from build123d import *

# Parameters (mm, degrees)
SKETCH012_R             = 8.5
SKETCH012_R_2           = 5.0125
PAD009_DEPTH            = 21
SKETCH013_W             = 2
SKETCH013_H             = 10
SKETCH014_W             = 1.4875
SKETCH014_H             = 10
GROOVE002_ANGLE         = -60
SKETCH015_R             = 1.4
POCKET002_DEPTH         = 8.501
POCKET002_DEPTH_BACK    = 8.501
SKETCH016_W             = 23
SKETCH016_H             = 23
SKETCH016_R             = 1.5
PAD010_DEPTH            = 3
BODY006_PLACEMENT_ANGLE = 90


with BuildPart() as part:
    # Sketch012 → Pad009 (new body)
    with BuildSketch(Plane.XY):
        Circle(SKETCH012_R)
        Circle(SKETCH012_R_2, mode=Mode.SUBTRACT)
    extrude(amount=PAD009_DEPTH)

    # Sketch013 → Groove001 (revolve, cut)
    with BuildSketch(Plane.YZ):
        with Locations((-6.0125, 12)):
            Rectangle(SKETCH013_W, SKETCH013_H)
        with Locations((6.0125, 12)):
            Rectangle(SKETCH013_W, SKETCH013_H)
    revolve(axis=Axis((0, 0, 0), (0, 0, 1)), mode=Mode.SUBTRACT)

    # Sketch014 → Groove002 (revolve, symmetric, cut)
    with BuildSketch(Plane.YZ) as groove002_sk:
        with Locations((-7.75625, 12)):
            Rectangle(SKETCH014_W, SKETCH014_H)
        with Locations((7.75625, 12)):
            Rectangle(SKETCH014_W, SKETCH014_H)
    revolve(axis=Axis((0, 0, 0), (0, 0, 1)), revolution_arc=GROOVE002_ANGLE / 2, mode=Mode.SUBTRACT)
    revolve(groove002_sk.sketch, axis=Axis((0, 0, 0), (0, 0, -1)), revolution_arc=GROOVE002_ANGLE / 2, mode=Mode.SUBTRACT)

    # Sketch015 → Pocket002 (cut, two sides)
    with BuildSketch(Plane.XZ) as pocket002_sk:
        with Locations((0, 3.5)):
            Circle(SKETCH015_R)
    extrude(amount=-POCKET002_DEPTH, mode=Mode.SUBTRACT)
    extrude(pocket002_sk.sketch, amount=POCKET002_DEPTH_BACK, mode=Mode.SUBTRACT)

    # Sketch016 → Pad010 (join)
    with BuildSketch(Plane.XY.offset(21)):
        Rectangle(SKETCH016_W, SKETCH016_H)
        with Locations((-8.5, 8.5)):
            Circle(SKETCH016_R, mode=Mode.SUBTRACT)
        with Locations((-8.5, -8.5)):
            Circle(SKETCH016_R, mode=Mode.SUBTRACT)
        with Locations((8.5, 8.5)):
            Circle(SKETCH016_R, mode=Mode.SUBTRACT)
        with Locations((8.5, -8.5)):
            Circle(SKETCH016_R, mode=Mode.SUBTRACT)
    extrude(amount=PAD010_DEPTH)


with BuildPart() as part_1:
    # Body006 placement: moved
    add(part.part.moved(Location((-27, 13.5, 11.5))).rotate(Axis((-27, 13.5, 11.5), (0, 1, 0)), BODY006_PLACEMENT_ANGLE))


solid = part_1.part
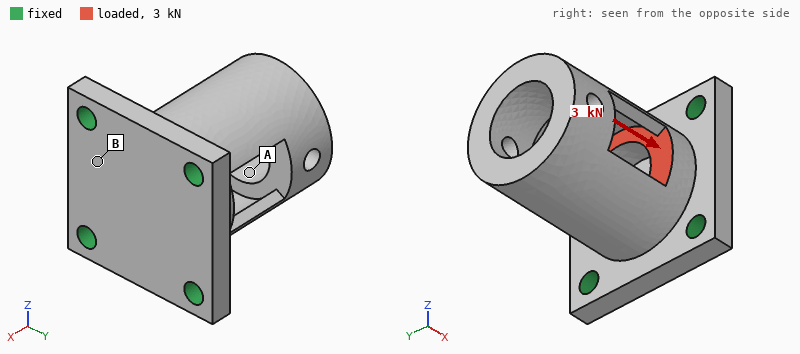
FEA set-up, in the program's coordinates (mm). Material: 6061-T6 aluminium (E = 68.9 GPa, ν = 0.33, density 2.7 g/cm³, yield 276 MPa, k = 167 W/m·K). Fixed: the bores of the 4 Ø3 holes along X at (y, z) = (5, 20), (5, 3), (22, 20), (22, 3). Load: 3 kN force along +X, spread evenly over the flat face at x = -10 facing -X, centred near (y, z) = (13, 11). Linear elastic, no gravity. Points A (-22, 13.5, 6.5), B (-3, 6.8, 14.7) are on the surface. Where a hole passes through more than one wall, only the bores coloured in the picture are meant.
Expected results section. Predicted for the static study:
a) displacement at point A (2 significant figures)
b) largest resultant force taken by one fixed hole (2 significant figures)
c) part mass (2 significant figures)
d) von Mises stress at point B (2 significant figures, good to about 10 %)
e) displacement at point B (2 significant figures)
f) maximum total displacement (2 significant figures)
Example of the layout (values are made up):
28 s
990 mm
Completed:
9.2 µm
790 N
9.6 g
37 MPa
9.7 µm
13 µm
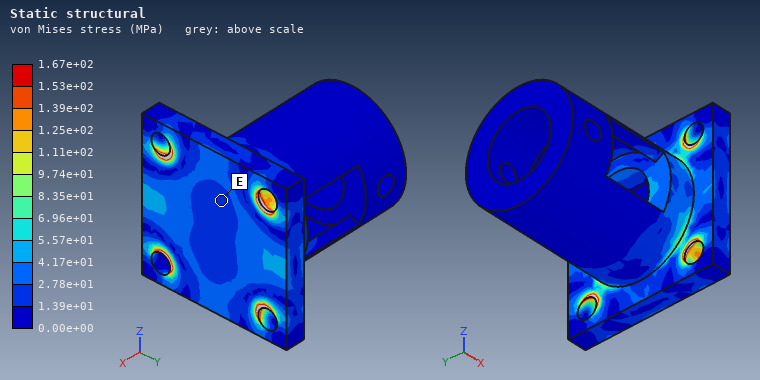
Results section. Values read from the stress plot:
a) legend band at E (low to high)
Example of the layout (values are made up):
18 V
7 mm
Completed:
1.39e+01 to 2.78e+01 MPa
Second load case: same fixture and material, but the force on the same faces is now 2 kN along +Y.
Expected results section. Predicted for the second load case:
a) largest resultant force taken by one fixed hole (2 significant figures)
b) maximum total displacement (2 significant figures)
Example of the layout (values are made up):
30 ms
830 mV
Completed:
630 N
18 µm
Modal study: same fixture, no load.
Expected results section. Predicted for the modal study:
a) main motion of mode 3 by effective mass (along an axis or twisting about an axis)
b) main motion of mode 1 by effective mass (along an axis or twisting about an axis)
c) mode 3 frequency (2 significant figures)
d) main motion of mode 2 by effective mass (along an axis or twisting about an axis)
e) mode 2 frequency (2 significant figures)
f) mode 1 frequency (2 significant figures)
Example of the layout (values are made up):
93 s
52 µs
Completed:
twisting about X
along Z
21 kHz
along Y
11 kHz
8400 Hz
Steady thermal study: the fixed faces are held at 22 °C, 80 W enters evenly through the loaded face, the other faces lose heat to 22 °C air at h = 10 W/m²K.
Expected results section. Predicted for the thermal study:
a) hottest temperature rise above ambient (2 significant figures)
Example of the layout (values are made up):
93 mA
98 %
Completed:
38 K
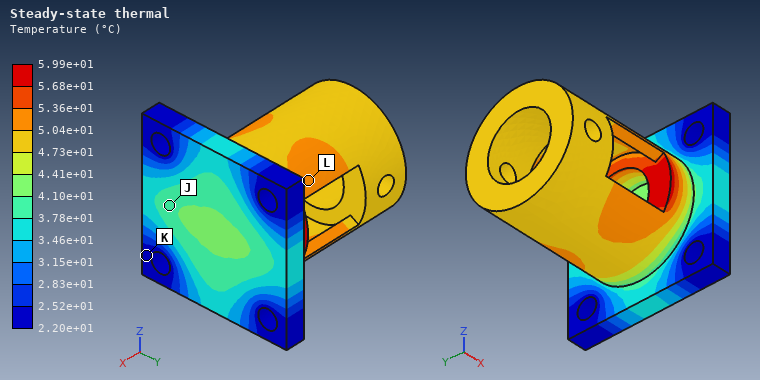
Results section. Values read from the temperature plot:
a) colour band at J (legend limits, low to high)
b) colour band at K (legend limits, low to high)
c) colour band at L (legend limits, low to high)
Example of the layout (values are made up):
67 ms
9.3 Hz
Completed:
3.78e+01 to 4.10e+01 °C
2.20e+01 to 2.52e+01 °C
5.04e+01 to 5.36e+01 °C
